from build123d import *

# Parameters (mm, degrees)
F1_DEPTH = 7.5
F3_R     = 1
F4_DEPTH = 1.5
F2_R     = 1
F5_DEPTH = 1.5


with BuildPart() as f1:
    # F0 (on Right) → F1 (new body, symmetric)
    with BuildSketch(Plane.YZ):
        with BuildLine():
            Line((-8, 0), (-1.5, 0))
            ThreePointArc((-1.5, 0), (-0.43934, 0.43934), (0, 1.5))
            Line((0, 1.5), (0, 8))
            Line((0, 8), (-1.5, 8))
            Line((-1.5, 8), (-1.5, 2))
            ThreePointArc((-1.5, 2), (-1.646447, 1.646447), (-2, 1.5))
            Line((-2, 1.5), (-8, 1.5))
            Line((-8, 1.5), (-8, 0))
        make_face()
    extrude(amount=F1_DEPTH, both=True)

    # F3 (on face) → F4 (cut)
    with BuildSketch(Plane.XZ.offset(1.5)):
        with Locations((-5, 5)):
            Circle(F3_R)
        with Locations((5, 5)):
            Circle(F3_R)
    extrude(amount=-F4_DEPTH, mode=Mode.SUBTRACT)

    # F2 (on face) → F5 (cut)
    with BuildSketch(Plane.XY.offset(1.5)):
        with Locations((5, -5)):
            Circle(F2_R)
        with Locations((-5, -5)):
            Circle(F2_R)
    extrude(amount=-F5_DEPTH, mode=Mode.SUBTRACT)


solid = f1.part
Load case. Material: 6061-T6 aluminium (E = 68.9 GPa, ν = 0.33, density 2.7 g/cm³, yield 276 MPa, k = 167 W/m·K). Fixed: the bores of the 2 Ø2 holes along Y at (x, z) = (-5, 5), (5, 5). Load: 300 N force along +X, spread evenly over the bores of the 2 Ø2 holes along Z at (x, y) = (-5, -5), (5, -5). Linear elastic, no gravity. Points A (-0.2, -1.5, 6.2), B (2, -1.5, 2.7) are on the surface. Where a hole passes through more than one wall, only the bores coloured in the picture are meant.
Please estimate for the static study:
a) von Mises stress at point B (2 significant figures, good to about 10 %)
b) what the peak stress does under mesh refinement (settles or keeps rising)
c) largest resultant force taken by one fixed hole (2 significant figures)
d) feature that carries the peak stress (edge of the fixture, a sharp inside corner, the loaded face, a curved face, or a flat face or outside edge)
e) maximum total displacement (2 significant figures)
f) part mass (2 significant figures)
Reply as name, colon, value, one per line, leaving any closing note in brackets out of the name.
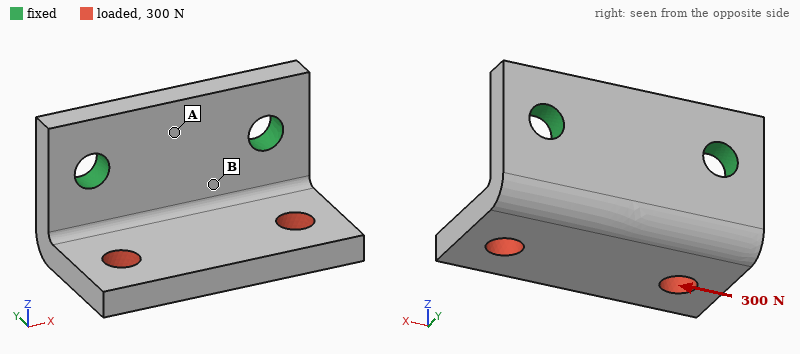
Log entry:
von Mises stress at point B: 70 MPa
what the peak stress does under mesh refinement: keeps rising
largest resultant force taken by one fixed hole: 220 N
feature that carries the peak stress: edge of the fixture
maximum total displacement: 32 µm
part mass: 0.81 g
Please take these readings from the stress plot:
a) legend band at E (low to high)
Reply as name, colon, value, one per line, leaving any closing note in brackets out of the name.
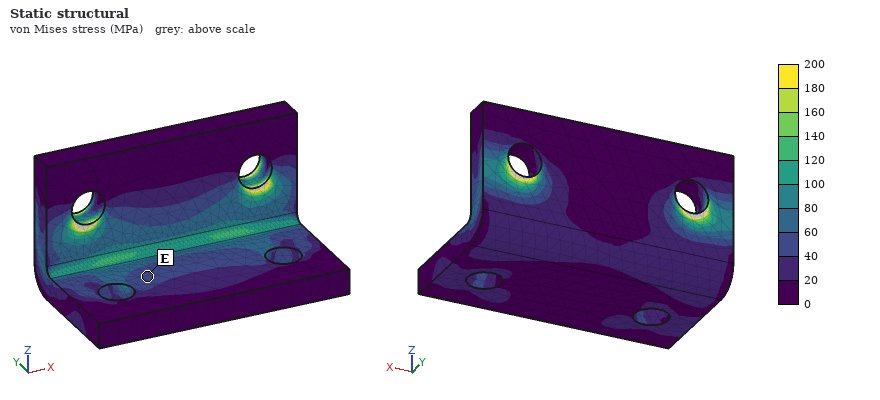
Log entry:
legend band at E: 40 to 60 MPa
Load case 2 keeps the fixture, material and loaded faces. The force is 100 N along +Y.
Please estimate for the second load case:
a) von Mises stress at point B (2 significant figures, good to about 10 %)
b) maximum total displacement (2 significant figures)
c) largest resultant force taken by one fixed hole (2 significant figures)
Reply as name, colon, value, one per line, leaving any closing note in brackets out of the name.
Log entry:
von Mises stress at point B: 24 MPa
maximum total displacement: 22 µm
largest resultant force taken by one fixed hole: 50 N
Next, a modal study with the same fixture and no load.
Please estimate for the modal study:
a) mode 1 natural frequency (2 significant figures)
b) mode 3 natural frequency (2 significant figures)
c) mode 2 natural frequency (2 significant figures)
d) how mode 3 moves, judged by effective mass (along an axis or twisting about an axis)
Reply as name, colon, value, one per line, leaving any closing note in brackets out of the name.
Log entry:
mode 1 natural frequency: 13 kHz
mode 3 natural frequency: 38 kHz
mode 2 natural frequency: 23 kHz
how mode 3 moves, judged by effective mass: along X
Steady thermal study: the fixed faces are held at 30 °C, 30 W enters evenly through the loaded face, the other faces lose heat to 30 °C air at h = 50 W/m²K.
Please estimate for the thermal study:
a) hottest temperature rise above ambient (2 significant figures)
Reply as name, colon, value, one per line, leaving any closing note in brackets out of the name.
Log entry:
hottest temperature rise above ambient: 76 K
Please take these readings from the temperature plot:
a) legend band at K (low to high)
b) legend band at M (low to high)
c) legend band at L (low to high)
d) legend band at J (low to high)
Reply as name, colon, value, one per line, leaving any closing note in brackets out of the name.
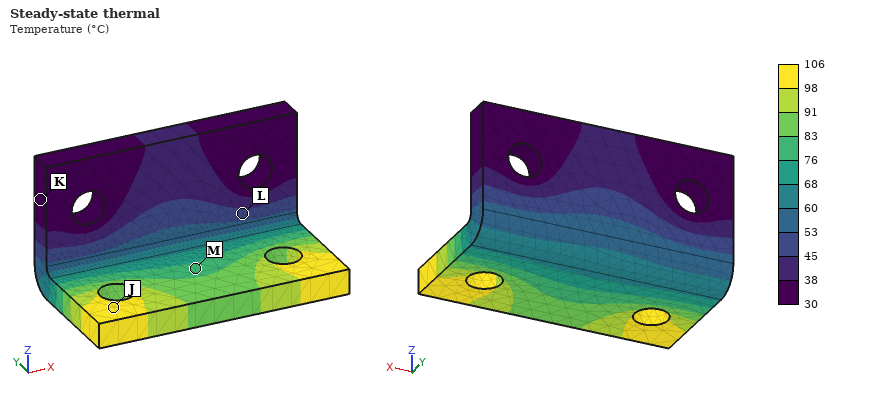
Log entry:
legend band at K: 30 to 38 °C
legend band at M: 76 to 83 °C
legend band at L: 45 to 53 °C
legend band at J: 98 to 106 °C
